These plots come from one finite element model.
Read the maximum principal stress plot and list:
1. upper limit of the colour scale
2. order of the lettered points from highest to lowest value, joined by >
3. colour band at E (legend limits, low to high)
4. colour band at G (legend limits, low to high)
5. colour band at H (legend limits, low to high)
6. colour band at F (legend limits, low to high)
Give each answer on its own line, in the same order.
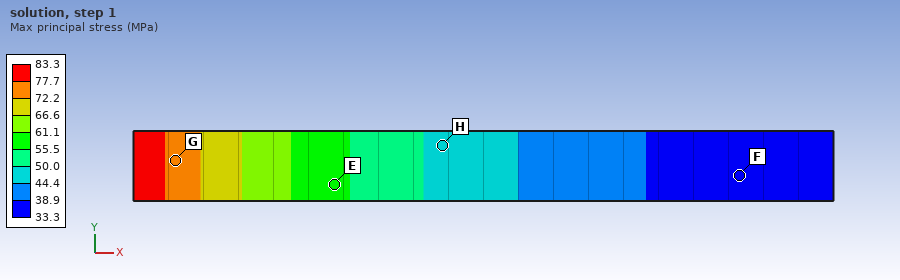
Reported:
83.3 MPa
G > E > H > F
55.5 to 61.1 MPa
72.2 to 77.7 MPa
44.4 to 50.0 MPa
33.3 to 38.9 MPa
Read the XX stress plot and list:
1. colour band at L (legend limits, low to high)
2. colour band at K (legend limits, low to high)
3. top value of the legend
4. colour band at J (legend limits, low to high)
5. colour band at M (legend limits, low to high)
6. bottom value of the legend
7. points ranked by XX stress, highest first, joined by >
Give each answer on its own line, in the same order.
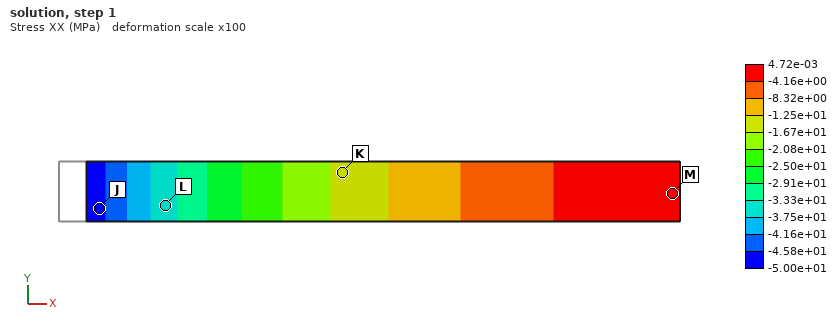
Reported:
-3.75e+01 to -3.33e+01 MPa
-1.67e+01 to -1.25e+01 MPa
4.72e-03 MPa
-5.00e+01 to -4.58e+01 MPa
-4.16e+00 to 4.72e-03 MPa
-5.00e+01 MPa
M > K > L > J
